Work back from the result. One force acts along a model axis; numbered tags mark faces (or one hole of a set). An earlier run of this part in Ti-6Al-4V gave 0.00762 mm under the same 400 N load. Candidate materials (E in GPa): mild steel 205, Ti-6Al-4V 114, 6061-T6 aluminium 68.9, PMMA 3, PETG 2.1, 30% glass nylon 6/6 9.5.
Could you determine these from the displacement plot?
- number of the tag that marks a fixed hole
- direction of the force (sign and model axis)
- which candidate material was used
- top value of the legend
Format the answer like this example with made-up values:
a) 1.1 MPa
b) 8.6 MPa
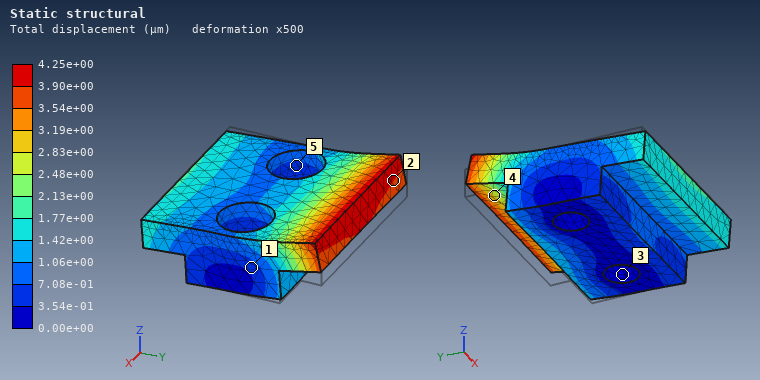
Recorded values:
a) 3
b) +Z
c) mild steel
d) 4.25e+00 µm
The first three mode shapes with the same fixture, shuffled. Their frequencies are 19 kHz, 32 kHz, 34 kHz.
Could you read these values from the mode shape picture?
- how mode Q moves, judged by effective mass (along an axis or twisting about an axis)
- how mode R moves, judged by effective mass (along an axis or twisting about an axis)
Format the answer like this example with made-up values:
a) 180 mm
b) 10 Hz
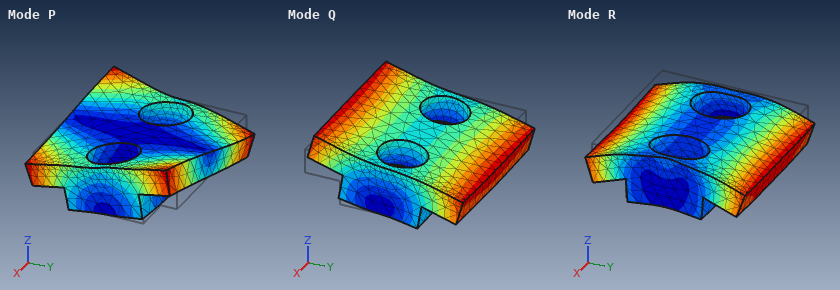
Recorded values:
a) along Y
b) along Z
